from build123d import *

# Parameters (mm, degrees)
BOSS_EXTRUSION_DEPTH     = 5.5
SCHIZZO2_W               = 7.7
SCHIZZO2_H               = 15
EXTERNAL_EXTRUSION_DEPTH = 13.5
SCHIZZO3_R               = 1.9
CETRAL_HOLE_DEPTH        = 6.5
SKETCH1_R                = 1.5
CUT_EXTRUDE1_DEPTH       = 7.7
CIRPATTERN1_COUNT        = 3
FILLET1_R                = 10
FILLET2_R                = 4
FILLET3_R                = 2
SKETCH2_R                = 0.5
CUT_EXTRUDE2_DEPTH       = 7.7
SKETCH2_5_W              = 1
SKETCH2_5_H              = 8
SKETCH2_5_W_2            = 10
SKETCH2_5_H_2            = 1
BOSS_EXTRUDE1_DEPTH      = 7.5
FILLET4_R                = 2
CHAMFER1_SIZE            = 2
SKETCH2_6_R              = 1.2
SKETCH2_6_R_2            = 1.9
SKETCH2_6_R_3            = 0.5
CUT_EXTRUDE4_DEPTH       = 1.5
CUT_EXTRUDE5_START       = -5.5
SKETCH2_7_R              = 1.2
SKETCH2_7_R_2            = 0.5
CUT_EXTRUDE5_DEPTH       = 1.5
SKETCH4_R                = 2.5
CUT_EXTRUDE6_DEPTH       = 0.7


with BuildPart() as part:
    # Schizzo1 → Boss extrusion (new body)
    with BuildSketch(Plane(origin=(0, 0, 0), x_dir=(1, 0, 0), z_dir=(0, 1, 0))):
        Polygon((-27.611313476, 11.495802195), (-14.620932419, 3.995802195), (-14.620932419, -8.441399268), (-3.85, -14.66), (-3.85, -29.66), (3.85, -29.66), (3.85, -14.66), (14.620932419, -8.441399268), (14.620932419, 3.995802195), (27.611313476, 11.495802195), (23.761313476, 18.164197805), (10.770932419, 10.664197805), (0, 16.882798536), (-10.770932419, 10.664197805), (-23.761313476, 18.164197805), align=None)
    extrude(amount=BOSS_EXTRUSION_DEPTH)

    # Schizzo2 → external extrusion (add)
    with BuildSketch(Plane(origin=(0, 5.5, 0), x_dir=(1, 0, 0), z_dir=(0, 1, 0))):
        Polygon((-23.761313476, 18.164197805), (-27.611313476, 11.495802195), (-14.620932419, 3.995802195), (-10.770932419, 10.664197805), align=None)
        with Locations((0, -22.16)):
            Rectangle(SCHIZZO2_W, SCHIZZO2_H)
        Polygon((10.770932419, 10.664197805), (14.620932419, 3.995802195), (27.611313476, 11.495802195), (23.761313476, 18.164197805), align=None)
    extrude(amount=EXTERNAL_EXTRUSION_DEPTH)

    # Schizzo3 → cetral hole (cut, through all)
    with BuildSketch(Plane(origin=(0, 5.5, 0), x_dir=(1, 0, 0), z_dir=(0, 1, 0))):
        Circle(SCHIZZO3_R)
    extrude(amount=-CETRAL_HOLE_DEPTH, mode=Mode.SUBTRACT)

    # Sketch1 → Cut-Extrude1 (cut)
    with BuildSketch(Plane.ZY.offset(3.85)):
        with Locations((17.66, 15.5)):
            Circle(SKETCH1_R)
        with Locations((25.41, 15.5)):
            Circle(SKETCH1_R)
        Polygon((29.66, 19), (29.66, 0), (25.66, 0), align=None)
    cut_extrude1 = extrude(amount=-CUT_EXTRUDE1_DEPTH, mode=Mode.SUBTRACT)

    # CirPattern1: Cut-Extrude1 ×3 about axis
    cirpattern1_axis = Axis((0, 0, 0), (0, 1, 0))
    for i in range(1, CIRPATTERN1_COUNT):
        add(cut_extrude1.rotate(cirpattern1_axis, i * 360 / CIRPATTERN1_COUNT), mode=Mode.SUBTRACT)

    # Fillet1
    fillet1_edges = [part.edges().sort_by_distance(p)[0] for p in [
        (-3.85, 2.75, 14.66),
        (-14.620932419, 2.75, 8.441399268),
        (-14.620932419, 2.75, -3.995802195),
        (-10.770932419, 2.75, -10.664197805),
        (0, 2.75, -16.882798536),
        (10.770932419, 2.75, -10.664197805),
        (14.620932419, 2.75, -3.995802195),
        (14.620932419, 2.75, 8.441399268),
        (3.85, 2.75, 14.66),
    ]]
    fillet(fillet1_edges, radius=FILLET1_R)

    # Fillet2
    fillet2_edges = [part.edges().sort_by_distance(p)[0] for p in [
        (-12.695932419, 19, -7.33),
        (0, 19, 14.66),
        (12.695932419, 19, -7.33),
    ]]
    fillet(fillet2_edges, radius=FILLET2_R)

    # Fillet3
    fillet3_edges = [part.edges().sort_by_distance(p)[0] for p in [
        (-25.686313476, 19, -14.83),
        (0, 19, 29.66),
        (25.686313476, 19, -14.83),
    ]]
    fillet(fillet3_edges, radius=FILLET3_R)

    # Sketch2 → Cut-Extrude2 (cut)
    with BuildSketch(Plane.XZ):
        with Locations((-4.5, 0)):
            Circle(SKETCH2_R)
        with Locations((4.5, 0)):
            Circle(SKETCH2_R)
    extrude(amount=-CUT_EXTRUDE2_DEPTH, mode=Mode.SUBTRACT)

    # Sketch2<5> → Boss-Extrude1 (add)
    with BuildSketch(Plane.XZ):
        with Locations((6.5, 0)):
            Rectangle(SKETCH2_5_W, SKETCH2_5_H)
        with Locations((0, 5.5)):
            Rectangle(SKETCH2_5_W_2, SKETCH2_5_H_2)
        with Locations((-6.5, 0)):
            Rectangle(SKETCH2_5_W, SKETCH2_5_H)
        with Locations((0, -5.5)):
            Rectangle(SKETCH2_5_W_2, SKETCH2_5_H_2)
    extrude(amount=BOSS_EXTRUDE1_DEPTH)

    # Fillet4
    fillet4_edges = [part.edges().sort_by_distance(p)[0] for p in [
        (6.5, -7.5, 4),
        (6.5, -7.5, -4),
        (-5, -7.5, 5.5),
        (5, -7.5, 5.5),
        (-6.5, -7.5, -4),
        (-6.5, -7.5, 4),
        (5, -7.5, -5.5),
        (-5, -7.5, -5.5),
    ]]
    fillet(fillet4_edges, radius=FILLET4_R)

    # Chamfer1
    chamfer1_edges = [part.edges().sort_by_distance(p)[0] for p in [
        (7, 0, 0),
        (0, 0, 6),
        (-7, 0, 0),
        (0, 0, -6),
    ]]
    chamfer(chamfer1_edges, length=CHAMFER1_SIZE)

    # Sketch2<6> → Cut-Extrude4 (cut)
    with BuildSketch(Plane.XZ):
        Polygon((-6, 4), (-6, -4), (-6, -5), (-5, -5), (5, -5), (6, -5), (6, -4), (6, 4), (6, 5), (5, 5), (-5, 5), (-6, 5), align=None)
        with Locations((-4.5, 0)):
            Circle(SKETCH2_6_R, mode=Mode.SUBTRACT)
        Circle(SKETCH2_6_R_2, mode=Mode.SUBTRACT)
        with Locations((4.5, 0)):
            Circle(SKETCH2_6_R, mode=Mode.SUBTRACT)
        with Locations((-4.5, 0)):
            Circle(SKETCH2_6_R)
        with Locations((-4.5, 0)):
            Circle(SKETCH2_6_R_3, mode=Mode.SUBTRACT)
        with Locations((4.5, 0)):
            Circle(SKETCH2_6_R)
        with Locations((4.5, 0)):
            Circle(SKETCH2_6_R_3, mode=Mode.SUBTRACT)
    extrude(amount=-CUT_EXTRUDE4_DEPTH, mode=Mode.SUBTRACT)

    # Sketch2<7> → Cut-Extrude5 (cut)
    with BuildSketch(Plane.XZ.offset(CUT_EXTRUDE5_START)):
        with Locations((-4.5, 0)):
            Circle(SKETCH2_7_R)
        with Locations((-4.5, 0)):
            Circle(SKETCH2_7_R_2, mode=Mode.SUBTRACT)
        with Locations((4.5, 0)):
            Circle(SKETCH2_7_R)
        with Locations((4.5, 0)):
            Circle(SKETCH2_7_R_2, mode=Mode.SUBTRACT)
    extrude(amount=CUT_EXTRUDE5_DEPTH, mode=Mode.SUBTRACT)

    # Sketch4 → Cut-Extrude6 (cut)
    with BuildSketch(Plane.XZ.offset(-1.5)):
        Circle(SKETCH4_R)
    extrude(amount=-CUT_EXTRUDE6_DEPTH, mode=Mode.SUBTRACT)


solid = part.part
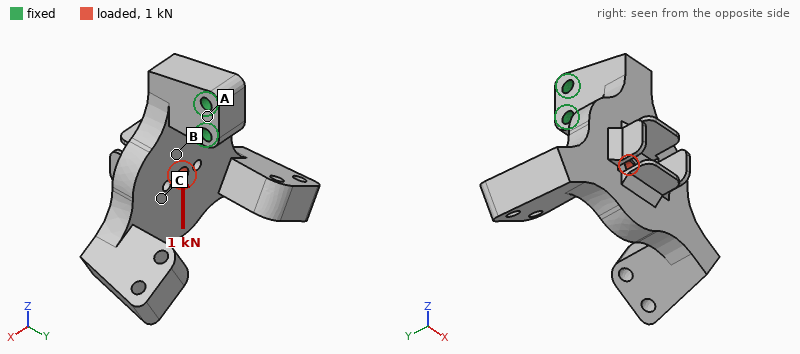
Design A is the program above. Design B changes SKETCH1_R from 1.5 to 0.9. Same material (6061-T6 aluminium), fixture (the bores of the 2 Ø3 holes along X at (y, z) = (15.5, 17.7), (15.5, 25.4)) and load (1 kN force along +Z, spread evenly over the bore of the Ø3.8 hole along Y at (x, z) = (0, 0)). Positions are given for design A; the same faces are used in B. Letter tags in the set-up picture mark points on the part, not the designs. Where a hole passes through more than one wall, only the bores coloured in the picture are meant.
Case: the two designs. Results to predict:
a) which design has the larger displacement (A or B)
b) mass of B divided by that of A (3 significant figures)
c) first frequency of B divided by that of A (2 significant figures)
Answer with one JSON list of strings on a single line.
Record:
["B", "1.02", "0.98"]
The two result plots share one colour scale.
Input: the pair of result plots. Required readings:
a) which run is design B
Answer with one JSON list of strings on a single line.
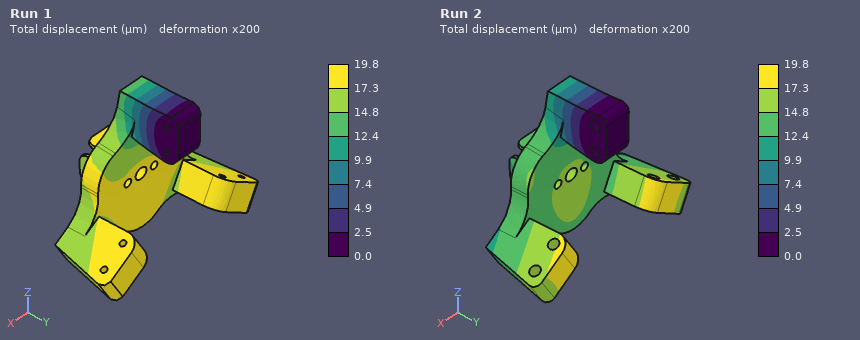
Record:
["Run 1"]
